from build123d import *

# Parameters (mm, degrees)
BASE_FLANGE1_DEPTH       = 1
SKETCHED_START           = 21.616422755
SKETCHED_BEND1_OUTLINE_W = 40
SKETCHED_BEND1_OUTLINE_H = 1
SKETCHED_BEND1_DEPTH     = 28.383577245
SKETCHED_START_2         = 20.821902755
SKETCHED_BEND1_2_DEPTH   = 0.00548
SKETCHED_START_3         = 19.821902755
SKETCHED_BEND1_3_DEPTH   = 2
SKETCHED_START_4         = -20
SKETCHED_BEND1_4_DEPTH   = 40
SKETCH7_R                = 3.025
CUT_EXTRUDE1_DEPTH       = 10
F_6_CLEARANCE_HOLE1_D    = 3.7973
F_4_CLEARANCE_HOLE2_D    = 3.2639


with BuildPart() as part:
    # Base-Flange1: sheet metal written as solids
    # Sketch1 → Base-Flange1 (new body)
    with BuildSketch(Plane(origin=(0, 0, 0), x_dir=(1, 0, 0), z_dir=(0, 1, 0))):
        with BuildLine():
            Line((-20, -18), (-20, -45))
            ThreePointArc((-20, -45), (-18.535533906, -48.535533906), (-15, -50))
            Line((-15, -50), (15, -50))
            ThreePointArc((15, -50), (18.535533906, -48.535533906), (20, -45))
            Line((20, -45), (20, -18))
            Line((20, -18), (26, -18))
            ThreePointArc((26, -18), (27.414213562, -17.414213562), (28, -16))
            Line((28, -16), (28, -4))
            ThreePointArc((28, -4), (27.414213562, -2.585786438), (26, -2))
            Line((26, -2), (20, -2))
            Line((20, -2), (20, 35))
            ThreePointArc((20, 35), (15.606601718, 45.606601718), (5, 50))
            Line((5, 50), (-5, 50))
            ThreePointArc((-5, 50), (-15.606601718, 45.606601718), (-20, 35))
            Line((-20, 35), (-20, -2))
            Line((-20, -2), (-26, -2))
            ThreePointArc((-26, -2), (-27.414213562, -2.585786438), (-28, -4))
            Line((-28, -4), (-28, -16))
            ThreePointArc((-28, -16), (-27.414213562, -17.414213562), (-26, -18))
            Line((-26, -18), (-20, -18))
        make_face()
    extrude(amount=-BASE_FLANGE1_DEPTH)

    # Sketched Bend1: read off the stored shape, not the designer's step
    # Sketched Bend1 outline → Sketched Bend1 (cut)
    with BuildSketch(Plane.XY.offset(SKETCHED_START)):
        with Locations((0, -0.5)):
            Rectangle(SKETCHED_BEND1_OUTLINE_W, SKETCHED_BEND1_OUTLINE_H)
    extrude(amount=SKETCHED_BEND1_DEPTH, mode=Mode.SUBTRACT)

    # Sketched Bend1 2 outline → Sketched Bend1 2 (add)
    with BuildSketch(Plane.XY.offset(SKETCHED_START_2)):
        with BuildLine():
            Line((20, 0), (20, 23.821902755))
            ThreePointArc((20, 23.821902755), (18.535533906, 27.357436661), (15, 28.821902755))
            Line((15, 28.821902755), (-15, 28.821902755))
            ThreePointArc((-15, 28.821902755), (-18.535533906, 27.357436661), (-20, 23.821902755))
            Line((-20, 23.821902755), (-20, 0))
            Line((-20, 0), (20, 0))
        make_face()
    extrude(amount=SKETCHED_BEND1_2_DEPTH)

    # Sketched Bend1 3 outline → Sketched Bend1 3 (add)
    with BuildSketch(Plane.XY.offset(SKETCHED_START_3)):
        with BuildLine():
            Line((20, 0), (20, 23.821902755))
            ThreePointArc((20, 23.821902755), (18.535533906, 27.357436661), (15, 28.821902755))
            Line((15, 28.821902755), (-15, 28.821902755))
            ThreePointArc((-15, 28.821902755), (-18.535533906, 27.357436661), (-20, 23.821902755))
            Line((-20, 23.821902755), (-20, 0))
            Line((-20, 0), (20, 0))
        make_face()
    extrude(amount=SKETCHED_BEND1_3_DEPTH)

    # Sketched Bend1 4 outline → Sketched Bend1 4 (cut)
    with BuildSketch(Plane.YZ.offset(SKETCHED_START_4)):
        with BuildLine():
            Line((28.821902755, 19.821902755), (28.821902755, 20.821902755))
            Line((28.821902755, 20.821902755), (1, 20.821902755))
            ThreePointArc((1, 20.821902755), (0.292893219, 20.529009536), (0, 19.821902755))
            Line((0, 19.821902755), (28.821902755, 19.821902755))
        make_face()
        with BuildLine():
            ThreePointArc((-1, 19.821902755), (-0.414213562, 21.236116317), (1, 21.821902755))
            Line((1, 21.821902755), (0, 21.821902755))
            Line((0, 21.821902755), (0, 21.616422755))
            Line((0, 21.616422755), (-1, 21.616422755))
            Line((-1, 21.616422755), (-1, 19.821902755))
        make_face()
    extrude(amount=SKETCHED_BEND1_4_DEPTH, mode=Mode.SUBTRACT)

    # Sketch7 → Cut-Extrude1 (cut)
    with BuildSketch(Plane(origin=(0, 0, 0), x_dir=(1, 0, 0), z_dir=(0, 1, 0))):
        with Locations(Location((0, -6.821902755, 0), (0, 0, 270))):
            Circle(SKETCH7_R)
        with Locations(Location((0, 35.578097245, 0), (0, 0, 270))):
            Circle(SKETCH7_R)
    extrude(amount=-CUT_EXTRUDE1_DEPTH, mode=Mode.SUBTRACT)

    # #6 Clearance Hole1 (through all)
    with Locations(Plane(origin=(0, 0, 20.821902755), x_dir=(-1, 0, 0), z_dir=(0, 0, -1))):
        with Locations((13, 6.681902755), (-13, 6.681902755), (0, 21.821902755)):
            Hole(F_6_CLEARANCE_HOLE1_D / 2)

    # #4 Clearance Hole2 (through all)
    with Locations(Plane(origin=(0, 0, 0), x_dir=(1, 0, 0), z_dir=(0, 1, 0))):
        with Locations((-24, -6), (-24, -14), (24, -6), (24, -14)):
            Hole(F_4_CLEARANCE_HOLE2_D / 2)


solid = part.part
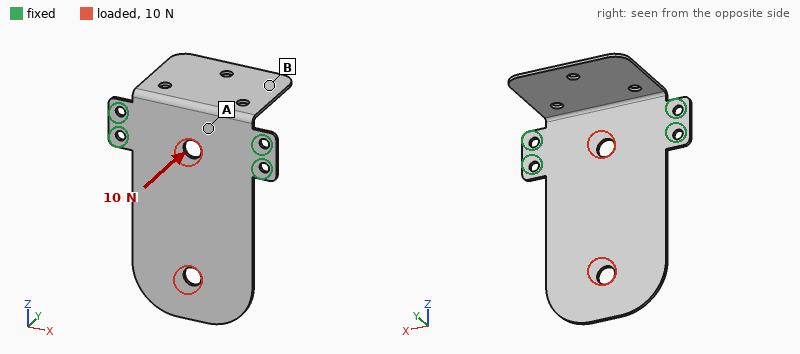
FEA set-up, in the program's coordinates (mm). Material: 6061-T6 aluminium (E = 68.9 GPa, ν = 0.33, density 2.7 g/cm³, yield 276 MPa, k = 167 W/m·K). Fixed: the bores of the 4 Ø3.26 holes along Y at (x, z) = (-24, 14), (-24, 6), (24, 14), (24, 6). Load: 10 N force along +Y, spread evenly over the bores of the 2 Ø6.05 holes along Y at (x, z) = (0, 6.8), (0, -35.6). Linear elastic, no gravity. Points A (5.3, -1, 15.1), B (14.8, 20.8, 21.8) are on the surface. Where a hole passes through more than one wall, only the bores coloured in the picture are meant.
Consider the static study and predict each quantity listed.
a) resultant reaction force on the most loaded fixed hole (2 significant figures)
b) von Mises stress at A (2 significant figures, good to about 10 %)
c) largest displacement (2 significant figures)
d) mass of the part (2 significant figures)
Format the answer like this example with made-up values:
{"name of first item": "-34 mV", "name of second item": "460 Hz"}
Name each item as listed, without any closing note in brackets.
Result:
{"resultant reaction force on the most loaded fixed hole": "12 N", "von Mises stress at A": "7.7 MPa", "largest displacement": "1.1 mm", "mass of the part": "11 g"}
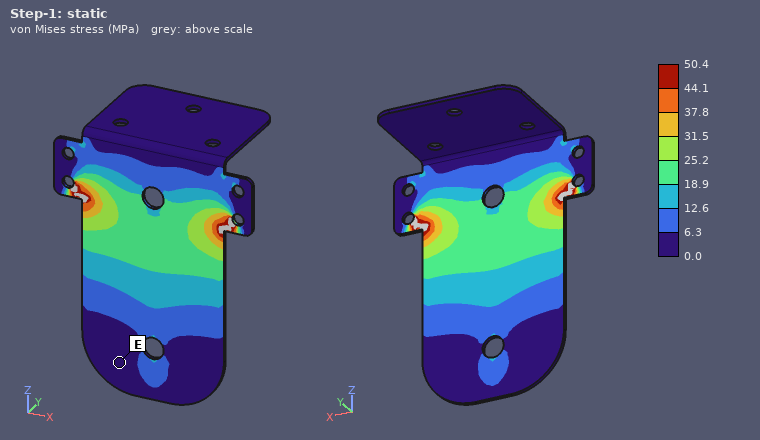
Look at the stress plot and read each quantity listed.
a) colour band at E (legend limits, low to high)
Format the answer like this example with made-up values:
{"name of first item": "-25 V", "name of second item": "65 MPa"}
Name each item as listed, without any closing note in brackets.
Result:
{"colour band at E": "0.0 to 6.3 MPa"}
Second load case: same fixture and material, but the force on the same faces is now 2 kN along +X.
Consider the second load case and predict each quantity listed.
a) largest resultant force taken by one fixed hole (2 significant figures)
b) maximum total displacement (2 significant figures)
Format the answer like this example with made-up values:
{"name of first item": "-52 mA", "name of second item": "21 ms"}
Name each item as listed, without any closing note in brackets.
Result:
{"largest resultant force taken by one fixed hole": "820 N", "maximum total displacement": "0.18 mm"}
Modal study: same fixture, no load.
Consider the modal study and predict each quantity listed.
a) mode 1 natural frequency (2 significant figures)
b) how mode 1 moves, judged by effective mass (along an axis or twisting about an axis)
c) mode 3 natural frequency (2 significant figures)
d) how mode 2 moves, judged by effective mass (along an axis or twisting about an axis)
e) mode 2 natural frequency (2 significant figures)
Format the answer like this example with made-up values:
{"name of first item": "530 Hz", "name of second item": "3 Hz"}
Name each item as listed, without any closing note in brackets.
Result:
{"mode 1 natural frequency": "240 Hz", "how mode 1 moves, judged by effective mass": "along Y", "mode 3 natural frequency": "930 Hz", "how mode 2 moves, judged by effective mass": "along Z", "mode 2 natural frequency": "650 Hz"}
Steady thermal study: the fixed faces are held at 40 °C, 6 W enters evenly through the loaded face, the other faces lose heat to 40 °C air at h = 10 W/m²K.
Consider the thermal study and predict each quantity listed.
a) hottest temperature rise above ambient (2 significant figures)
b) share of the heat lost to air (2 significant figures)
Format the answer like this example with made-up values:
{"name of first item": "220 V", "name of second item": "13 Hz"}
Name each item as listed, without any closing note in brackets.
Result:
{"hottest temperature rise above ambient": "28 K", "share of the heat lost to air": "17 %"}
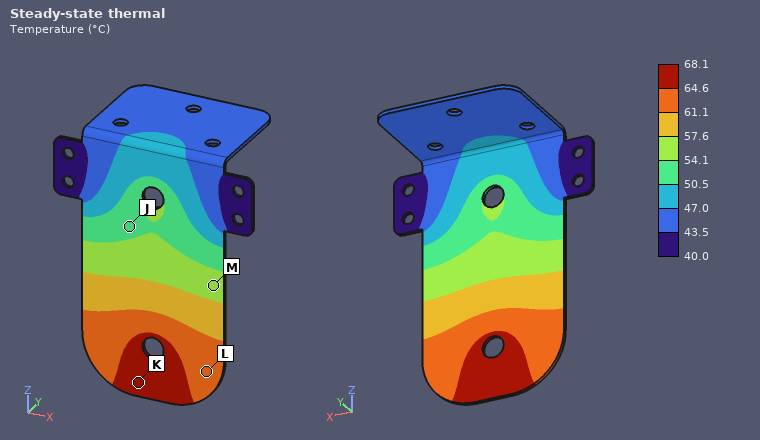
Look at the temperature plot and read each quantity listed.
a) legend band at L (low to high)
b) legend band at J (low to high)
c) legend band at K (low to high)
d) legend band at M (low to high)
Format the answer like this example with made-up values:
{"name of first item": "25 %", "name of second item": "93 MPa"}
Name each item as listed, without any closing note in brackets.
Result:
{"legend band at L": "61.1 to 64.6 °C", "legend band at J": "50.5 to 54.1 °C", "legend band at K": "64.6 to 68.1 °C", "legend band at M": "54.1 to 57.6 °C"}
